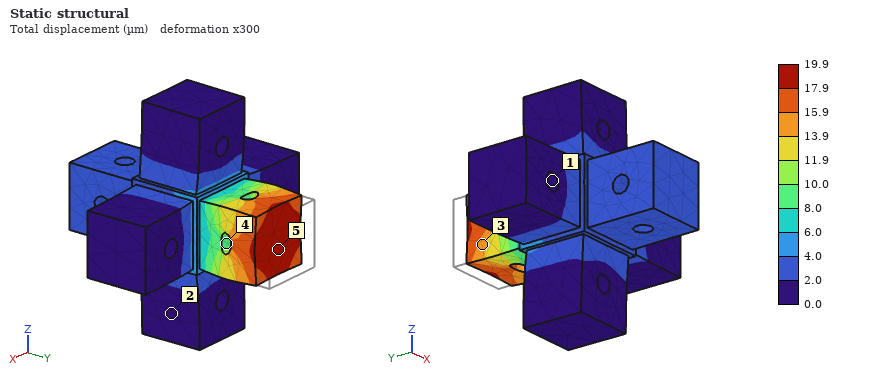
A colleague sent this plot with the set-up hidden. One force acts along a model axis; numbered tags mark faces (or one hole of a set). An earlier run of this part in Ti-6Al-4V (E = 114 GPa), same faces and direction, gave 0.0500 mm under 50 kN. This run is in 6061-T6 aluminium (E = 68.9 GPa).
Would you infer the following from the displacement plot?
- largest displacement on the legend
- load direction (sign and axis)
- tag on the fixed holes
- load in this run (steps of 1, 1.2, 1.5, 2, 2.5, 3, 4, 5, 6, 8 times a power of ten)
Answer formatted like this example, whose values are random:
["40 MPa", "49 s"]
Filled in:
["19.9 µm", "-Y", "1", "12 kN"]
